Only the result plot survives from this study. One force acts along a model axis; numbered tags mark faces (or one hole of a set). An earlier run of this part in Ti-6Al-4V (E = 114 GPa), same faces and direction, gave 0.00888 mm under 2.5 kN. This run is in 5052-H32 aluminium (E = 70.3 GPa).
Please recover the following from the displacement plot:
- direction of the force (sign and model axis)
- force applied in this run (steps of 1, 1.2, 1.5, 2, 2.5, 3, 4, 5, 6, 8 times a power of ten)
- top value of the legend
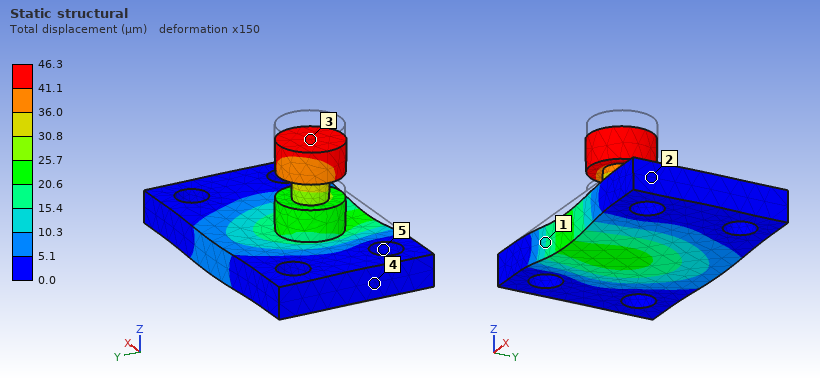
-Z
8 kN
46.3 µm
